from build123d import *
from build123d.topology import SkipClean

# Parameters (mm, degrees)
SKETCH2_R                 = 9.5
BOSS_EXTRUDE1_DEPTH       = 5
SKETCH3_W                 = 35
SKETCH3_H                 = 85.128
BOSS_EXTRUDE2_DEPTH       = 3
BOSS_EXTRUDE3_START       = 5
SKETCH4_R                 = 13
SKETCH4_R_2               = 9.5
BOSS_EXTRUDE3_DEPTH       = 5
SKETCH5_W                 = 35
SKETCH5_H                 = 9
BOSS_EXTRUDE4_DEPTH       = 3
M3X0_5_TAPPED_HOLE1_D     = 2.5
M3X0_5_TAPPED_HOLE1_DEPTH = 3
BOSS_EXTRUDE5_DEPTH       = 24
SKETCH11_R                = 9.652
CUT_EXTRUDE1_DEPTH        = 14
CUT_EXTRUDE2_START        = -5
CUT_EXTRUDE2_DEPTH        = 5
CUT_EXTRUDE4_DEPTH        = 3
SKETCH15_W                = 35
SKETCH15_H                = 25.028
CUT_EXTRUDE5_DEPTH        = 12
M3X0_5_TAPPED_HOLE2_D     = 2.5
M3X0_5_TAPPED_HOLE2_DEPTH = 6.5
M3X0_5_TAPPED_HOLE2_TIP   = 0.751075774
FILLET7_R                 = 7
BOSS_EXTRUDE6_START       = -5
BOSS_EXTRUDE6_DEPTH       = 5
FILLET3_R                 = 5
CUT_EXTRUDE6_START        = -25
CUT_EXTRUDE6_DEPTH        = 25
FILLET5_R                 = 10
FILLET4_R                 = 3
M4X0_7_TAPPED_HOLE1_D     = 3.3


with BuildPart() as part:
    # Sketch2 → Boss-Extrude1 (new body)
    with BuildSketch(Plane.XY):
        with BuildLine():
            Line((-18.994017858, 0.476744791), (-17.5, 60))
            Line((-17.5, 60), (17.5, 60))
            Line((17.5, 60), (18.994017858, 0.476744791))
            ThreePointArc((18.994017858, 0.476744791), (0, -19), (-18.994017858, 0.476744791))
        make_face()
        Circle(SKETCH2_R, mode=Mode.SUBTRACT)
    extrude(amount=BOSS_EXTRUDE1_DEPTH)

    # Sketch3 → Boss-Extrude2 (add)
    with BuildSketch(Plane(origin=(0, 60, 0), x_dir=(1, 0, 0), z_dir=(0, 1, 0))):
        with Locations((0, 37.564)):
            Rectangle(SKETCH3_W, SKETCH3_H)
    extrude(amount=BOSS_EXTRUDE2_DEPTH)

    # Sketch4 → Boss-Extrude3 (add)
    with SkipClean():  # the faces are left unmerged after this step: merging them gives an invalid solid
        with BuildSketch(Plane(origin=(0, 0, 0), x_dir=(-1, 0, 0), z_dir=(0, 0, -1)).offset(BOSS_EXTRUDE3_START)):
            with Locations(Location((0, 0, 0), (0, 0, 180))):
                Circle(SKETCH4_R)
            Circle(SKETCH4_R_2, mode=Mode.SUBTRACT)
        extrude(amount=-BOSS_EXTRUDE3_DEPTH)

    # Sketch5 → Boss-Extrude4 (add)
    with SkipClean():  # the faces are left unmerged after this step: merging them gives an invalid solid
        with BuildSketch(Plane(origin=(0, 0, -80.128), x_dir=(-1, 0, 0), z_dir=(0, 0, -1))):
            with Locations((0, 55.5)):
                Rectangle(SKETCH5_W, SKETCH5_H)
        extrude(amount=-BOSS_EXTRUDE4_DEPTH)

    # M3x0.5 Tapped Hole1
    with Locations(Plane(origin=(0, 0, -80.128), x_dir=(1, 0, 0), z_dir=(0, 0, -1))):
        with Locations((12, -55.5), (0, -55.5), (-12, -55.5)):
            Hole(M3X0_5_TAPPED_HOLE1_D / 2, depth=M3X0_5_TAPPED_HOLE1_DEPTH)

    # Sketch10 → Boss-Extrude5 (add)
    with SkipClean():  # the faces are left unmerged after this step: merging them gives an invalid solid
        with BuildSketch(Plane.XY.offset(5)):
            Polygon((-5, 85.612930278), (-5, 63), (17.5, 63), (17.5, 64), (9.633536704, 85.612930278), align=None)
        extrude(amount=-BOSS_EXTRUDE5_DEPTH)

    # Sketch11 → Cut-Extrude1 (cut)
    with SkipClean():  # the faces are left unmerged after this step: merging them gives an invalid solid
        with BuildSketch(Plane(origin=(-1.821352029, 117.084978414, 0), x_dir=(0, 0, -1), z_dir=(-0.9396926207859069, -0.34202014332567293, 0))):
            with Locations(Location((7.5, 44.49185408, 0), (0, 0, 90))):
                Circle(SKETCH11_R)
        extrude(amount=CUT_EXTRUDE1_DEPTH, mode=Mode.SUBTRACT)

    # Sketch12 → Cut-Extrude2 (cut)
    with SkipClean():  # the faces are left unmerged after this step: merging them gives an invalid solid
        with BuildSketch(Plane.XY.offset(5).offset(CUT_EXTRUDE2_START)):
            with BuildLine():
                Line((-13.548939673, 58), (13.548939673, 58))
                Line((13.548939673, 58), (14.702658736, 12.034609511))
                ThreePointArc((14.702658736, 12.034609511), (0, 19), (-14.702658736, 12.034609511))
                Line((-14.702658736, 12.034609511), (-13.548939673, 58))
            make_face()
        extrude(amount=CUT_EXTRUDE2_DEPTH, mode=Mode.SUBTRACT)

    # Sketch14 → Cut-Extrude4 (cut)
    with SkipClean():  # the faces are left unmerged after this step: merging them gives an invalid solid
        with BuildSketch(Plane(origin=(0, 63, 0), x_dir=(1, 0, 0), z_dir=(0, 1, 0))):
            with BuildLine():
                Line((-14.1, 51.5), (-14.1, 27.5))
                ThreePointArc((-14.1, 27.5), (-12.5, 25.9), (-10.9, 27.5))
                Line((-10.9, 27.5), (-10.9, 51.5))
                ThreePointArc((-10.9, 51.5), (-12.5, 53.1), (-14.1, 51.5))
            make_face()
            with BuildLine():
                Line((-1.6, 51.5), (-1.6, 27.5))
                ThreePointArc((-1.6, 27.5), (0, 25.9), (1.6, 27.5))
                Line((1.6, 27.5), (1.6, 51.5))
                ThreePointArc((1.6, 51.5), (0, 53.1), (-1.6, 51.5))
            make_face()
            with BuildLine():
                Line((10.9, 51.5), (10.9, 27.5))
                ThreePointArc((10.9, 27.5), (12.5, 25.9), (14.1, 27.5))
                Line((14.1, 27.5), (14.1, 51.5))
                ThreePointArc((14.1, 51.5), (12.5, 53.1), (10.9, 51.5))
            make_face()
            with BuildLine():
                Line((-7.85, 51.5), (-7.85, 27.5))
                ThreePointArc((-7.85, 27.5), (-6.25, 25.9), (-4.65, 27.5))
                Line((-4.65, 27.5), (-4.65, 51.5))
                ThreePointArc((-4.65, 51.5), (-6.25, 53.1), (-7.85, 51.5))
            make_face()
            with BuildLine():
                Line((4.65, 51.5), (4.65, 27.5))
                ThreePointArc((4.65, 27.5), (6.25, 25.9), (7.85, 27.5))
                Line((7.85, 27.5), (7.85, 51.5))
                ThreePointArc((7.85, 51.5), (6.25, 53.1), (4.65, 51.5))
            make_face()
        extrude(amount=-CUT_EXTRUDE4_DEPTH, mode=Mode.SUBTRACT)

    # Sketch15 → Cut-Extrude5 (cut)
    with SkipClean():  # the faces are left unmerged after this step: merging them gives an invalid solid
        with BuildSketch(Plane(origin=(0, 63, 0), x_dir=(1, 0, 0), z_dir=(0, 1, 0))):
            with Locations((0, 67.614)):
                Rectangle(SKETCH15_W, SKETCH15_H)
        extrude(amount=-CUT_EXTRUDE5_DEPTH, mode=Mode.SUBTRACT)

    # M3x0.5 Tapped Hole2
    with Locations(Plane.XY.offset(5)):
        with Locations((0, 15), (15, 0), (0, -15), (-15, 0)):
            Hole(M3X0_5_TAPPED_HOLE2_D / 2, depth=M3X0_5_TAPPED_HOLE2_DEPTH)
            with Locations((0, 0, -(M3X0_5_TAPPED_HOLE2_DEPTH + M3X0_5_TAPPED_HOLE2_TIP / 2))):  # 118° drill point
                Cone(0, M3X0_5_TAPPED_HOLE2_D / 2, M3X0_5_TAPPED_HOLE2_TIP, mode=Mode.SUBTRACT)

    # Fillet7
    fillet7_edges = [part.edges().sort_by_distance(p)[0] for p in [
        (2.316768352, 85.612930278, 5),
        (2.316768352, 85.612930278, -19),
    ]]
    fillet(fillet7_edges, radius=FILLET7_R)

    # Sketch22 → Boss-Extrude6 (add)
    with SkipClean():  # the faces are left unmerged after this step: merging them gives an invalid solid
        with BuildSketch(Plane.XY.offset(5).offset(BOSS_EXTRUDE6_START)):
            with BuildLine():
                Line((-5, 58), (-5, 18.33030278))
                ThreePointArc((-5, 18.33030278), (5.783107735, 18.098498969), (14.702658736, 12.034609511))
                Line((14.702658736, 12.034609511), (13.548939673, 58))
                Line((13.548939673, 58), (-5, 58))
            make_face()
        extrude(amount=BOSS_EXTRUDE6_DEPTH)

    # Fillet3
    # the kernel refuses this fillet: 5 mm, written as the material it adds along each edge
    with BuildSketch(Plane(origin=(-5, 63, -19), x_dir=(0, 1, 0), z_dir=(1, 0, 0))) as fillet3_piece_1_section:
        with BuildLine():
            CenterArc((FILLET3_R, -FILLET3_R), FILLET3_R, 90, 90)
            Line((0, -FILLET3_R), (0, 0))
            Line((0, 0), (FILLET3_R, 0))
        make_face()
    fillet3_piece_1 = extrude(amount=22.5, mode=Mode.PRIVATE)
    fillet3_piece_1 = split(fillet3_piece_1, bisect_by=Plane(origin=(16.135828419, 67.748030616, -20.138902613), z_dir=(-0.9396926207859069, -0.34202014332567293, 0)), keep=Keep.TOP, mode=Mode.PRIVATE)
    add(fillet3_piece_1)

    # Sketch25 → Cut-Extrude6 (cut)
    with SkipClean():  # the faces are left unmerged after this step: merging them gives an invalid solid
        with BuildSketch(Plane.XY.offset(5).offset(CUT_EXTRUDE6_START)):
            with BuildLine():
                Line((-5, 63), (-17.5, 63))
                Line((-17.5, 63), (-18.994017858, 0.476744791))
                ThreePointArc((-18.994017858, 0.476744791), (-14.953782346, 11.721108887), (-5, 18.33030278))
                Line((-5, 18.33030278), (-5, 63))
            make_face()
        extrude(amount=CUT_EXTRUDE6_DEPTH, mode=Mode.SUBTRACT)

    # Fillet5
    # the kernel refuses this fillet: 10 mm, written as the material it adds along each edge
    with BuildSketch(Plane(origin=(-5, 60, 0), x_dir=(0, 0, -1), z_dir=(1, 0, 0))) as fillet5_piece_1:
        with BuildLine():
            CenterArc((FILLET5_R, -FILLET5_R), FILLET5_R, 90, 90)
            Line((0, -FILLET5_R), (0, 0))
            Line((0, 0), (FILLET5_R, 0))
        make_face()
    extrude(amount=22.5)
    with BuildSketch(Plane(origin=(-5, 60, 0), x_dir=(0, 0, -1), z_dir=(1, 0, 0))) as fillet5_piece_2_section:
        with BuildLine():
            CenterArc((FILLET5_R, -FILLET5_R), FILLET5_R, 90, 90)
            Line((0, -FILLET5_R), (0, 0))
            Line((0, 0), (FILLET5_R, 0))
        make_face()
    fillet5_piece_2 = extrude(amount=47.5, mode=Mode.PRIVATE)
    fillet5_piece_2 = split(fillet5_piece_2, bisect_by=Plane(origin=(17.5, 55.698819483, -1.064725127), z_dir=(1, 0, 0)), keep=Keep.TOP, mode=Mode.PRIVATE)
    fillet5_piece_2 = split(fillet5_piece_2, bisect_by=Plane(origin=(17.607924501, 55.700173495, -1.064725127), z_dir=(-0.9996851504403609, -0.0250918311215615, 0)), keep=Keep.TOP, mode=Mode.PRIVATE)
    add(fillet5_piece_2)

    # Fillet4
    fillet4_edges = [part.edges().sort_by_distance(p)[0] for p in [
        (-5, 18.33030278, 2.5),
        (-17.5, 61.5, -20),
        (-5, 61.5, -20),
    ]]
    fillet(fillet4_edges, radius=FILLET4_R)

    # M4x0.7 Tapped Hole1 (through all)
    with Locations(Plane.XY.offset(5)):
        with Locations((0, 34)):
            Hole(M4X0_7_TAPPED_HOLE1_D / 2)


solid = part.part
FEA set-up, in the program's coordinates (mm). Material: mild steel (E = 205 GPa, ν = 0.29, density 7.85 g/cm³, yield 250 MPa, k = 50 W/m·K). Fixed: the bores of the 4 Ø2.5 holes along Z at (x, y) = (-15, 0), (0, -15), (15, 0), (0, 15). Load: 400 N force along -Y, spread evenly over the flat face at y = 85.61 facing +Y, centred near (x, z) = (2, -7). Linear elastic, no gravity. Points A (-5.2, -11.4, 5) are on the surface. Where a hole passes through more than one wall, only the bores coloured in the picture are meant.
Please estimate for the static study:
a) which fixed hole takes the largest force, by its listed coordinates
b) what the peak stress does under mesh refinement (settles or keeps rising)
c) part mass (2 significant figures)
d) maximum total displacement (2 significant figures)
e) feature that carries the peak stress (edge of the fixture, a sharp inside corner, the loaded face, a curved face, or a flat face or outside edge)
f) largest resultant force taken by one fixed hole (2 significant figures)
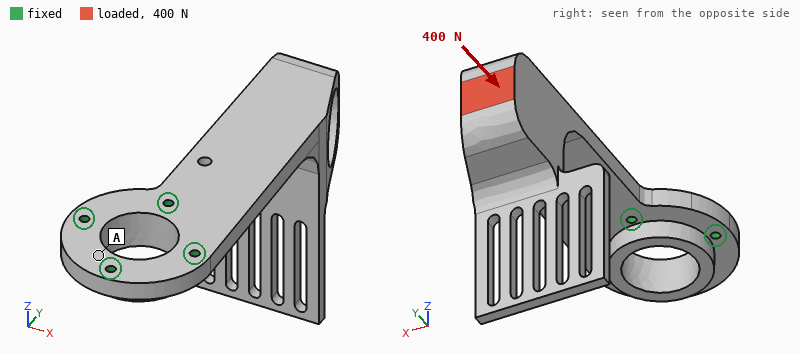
(0, 15)
keeps rising
160 g
0.22 mm
edge of the fixture
290 N
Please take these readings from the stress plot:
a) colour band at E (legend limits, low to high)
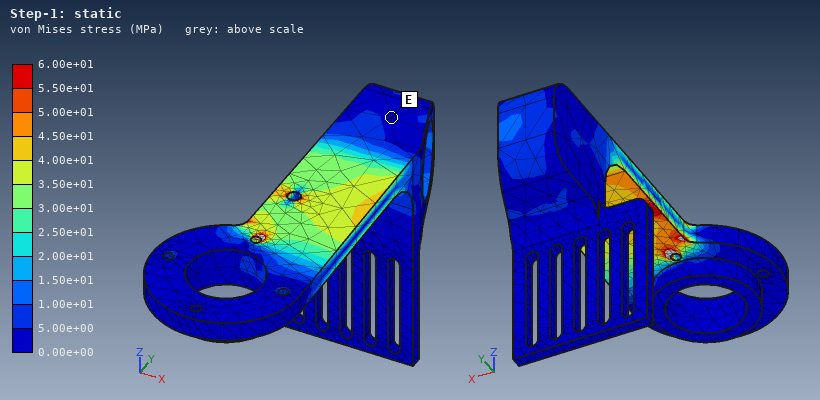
0.00e+00 to 5.00e+00 MPa
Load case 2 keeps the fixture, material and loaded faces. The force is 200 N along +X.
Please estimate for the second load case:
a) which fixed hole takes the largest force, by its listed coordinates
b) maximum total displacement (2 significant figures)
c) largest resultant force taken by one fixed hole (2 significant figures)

(15, 0)
85 µm
710 N
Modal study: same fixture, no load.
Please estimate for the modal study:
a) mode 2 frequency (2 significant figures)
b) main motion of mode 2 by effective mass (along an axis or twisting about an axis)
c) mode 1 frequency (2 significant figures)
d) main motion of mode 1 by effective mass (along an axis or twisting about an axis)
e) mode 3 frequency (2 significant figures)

890 Hz
along X
430 Hz
along Z
1600 Hz
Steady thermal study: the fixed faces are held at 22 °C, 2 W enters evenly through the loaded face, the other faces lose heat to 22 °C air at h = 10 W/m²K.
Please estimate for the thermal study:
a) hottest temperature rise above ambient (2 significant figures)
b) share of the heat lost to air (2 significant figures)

16 K
42 %
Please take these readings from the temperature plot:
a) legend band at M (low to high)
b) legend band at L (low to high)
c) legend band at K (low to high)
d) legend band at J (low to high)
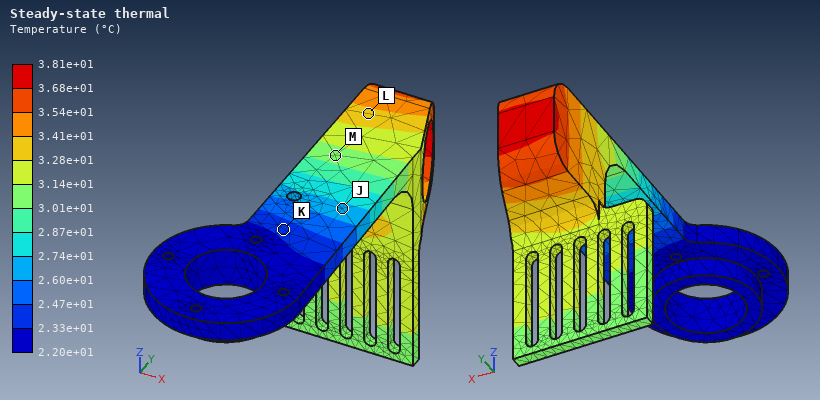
3.01e+01 to 3.14e+01 °C
3.28e+01 to 3.41e+01 °C
2.33e+01 to 2.47e+01 °C
2.60e+01 to 2.74e+01 °C
